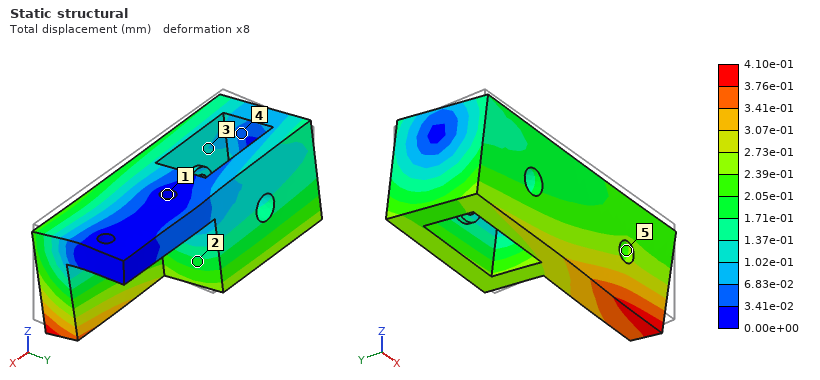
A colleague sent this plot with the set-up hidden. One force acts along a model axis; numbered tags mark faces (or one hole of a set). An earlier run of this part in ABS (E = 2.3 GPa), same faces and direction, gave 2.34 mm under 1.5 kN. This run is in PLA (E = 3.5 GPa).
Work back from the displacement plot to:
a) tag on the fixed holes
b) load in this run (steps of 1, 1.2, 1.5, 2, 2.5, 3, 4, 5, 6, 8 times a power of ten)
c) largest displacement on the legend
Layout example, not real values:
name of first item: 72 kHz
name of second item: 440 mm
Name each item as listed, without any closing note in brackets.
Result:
tag on the fixed holes: 1
load in this run: 400 N
largest displacement on the legend: 4.10e-01 mm
